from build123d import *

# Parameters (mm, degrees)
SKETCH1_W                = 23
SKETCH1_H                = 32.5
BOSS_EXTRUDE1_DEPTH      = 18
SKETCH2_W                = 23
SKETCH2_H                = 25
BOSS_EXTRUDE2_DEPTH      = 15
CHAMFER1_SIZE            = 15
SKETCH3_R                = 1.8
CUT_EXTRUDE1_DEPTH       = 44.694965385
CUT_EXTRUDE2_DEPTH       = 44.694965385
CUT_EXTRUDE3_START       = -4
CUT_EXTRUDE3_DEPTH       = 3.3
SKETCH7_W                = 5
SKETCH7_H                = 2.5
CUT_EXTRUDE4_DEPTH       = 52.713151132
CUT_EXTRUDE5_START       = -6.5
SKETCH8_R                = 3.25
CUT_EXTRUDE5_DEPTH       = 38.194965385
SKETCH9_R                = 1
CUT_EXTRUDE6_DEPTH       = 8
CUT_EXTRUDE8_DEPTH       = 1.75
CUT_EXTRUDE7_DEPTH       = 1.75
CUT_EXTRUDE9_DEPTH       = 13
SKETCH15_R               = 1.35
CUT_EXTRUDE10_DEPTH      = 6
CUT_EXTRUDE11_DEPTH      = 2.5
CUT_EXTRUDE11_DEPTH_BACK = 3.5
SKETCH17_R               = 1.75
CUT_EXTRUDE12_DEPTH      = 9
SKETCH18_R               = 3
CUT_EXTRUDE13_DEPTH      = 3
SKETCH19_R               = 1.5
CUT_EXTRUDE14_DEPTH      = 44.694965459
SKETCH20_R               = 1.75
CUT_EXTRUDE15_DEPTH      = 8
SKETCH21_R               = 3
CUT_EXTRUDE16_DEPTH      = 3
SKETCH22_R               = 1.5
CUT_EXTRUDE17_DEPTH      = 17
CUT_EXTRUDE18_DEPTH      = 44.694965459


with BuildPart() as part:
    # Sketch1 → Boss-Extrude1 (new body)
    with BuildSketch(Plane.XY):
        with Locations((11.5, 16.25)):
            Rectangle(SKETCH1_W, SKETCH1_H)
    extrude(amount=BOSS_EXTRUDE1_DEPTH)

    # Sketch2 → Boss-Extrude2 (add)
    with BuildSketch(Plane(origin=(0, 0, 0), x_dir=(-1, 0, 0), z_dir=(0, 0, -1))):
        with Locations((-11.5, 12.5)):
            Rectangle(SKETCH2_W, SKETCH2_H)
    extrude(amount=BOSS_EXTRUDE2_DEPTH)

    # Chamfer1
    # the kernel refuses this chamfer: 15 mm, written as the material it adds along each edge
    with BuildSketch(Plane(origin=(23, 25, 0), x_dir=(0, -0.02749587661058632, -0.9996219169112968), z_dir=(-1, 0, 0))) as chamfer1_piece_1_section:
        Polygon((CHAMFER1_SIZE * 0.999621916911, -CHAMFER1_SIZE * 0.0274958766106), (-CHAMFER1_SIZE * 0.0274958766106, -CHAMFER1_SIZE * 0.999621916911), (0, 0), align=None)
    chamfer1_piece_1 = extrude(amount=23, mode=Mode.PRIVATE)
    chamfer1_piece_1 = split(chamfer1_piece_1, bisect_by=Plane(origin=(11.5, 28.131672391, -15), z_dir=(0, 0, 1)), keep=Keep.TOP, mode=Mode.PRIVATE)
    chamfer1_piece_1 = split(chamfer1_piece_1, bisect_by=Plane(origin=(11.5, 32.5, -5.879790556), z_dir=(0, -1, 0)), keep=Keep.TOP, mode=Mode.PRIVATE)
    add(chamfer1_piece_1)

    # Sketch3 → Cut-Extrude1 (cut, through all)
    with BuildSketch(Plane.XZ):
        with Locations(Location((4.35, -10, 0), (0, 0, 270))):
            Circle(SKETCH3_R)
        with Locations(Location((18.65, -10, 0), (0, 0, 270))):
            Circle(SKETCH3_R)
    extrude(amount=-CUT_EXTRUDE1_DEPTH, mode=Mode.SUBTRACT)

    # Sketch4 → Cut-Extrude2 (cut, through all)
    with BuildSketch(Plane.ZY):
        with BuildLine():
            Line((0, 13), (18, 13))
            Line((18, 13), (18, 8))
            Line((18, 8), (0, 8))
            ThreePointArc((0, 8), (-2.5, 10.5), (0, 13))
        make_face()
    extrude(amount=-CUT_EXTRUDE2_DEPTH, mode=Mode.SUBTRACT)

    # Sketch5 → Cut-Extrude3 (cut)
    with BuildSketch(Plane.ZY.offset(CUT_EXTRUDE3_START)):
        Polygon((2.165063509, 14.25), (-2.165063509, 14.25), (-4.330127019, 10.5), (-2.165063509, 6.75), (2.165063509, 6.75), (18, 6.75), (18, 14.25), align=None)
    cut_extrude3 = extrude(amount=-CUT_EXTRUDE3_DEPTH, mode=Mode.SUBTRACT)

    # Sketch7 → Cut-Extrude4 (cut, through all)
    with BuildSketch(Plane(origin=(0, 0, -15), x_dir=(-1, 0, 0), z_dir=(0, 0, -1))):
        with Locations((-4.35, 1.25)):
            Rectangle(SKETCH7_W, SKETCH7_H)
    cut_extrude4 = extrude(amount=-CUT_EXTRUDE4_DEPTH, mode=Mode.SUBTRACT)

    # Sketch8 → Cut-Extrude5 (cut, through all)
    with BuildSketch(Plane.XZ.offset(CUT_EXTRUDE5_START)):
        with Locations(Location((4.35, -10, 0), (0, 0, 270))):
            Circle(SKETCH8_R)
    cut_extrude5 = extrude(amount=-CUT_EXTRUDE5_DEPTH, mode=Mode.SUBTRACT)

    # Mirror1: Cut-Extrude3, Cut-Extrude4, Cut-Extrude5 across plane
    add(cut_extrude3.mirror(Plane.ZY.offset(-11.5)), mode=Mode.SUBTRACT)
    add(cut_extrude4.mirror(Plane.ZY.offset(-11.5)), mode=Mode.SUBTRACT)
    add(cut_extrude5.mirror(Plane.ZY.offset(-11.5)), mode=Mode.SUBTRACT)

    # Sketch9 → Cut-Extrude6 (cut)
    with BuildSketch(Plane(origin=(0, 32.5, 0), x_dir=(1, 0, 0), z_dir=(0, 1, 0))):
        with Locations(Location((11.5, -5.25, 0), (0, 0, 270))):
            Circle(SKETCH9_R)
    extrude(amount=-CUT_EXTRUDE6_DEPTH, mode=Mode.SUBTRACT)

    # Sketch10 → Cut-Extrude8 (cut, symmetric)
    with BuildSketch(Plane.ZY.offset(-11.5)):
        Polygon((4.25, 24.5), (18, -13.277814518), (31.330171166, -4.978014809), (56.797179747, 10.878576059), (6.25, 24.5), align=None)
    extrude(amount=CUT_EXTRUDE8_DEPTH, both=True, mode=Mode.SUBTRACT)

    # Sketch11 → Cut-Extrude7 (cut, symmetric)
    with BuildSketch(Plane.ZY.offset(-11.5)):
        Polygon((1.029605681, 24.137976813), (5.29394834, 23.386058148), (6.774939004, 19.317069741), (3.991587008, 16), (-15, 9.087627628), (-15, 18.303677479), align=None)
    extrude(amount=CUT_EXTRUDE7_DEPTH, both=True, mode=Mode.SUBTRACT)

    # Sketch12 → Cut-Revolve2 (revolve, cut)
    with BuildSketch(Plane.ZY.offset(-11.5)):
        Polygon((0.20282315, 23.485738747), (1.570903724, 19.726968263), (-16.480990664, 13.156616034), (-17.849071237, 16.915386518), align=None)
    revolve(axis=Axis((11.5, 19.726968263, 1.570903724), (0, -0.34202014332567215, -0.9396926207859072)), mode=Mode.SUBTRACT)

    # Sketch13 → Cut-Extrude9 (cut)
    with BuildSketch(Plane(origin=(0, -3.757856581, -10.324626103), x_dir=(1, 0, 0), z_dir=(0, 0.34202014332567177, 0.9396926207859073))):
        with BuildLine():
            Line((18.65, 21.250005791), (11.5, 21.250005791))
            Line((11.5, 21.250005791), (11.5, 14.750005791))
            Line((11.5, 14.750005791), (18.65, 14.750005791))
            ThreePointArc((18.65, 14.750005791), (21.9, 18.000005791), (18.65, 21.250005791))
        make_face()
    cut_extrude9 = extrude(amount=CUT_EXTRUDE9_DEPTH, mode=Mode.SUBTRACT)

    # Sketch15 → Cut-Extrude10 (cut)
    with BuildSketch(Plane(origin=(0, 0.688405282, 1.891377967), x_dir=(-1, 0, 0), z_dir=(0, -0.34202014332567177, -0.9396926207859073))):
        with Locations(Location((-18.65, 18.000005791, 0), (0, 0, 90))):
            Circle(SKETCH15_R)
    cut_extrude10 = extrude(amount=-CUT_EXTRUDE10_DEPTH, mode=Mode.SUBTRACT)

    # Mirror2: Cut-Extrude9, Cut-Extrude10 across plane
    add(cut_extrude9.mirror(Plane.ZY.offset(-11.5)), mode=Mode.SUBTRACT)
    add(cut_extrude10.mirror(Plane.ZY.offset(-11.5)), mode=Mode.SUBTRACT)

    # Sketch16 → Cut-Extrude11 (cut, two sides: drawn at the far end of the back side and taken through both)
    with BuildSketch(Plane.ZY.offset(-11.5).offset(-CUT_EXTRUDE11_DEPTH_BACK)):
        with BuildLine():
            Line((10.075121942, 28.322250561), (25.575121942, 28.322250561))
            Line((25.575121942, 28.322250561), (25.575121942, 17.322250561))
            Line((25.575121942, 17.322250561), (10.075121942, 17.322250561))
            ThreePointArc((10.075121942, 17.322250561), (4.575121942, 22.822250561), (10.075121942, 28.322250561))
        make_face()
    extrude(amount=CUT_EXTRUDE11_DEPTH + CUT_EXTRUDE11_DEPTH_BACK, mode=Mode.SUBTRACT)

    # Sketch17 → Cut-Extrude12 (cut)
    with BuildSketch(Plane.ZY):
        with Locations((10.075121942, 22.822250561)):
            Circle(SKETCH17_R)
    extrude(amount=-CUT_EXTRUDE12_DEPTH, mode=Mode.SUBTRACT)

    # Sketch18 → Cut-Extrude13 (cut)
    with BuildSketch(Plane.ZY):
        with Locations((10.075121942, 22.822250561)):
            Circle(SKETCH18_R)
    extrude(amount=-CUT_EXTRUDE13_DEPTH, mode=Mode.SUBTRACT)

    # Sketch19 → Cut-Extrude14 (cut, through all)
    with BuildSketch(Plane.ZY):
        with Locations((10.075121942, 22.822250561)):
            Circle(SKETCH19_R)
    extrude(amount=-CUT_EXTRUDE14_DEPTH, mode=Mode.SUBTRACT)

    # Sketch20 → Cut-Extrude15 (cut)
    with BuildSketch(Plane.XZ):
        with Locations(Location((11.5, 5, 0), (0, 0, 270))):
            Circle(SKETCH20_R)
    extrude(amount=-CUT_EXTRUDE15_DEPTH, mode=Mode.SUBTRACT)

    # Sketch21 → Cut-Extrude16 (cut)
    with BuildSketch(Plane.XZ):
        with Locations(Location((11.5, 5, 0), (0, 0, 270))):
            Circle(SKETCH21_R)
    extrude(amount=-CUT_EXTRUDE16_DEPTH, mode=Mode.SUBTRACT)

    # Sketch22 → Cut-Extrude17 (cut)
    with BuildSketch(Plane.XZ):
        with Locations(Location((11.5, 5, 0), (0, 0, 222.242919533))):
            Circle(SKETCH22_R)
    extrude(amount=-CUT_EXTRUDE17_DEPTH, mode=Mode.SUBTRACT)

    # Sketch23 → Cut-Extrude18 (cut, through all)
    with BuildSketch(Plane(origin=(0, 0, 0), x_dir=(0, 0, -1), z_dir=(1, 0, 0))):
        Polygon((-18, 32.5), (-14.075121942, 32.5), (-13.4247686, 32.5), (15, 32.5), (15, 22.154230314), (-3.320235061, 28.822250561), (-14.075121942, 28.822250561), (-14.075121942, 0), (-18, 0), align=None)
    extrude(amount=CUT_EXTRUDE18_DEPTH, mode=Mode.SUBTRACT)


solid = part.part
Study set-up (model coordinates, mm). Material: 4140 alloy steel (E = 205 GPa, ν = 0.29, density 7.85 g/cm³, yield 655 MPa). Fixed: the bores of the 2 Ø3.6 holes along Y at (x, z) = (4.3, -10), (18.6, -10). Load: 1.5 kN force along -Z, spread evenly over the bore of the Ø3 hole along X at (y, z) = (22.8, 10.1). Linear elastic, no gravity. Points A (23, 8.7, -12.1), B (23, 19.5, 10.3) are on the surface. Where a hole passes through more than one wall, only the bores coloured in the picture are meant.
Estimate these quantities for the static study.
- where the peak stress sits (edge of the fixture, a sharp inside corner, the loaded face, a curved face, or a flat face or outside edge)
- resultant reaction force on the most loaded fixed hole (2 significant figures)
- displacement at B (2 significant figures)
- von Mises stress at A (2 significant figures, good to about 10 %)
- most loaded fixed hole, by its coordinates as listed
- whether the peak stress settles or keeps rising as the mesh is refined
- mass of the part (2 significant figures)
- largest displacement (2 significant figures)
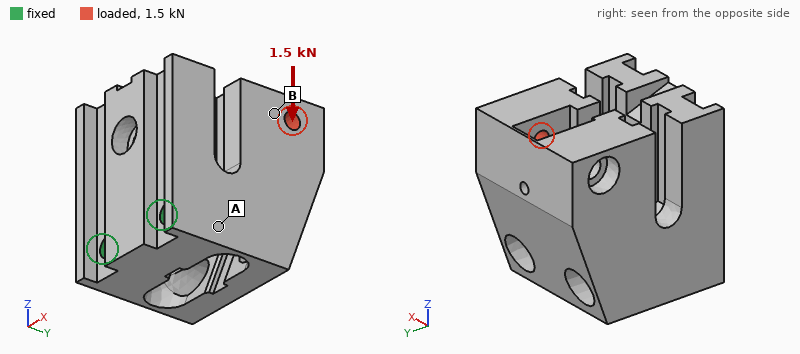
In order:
edge of the fixture
1.4 kN
59 µm
91 MPa
(18.6, -10)
keeps rising
87 g
83 µm
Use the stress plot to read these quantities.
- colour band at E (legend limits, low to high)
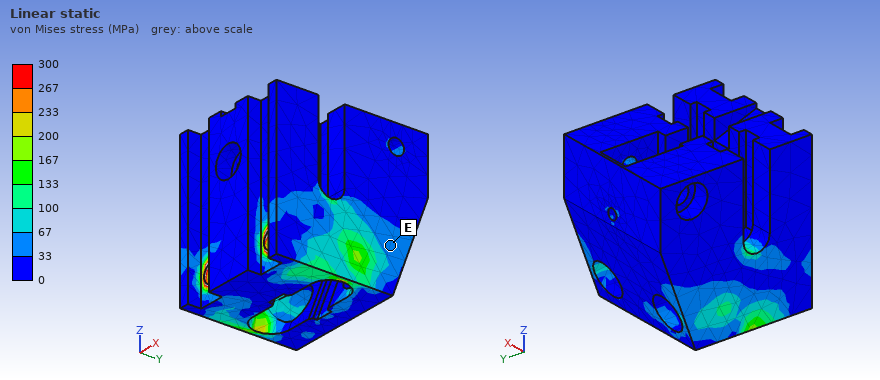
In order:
33 to 67 MPa
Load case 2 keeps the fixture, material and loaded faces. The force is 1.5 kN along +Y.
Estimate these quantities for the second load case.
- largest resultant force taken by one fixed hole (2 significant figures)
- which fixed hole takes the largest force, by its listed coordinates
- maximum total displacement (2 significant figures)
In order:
1.4 kN
(18.6, -10)
0.10 mm
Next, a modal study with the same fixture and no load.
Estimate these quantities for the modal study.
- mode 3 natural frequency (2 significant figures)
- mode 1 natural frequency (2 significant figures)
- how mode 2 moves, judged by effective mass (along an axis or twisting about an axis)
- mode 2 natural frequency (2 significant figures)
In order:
9700 Hz
3600 Hz
along X
8200 Hz
